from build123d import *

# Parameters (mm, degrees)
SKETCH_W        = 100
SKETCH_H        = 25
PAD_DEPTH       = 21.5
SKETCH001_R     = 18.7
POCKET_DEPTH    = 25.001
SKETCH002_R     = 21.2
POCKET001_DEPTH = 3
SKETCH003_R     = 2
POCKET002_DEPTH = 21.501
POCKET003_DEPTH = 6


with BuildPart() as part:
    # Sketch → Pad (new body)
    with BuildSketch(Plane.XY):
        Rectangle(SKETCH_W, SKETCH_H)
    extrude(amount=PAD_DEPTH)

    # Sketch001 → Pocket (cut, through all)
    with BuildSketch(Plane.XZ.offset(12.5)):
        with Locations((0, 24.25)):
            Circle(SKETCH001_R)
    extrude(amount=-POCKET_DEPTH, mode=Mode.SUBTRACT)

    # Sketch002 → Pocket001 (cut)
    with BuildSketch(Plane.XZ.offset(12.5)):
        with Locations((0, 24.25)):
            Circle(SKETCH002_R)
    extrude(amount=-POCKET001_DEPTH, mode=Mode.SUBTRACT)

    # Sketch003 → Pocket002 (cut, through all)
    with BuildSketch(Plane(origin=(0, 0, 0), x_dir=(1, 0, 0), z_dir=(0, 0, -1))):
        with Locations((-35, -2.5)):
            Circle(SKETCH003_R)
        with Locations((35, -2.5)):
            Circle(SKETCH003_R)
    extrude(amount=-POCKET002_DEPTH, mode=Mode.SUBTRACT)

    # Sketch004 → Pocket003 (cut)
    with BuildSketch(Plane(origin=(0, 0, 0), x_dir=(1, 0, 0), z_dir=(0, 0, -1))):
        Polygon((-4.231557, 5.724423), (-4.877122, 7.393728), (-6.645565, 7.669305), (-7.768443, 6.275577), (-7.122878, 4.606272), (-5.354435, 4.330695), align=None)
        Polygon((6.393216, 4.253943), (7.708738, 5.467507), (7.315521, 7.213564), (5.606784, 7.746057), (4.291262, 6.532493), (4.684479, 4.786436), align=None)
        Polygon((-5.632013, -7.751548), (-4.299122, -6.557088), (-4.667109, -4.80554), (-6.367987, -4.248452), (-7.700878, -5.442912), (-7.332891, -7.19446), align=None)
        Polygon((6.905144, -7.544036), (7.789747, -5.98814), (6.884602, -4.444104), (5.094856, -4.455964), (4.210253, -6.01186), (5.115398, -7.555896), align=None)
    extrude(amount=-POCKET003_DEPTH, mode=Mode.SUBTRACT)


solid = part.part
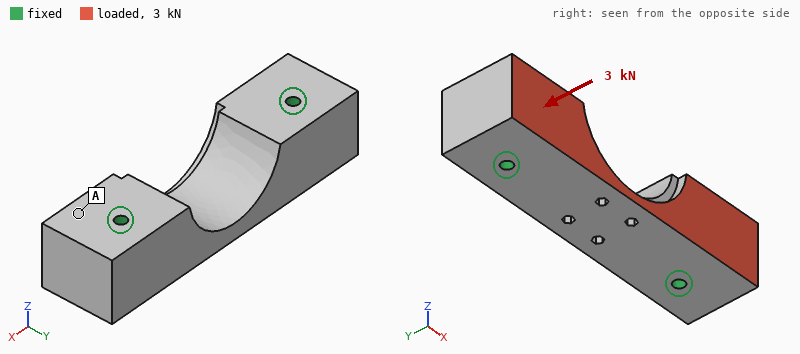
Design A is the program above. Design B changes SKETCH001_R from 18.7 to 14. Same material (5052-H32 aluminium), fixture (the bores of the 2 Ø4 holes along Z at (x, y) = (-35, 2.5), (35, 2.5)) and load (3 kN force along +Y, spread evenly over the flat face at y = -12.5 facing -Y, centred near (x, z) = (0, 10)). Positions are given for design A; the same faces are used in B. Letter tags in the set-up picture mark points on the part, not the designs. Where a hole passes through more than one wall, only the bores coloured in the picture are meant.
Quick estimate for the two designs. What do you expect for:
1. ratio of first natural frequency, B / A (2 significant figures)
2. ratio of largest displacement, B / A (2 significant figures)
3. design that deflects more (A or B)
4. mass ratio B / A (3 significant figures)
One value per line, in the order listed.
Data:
0.99
0.80
A
1.11
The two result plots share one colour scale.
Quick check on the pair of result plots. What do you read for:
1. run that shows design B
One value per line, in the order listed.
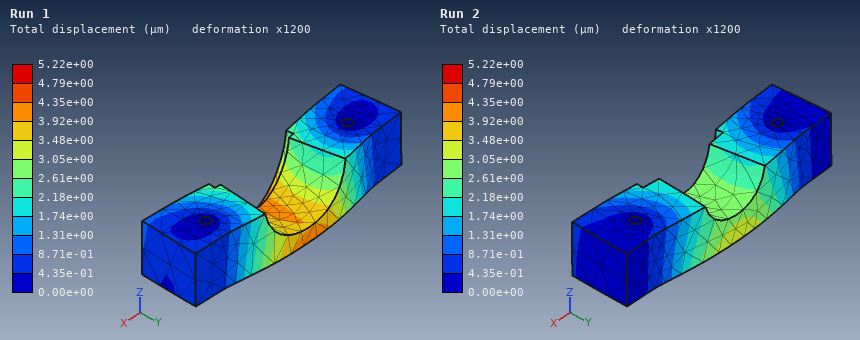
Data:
Run 2
